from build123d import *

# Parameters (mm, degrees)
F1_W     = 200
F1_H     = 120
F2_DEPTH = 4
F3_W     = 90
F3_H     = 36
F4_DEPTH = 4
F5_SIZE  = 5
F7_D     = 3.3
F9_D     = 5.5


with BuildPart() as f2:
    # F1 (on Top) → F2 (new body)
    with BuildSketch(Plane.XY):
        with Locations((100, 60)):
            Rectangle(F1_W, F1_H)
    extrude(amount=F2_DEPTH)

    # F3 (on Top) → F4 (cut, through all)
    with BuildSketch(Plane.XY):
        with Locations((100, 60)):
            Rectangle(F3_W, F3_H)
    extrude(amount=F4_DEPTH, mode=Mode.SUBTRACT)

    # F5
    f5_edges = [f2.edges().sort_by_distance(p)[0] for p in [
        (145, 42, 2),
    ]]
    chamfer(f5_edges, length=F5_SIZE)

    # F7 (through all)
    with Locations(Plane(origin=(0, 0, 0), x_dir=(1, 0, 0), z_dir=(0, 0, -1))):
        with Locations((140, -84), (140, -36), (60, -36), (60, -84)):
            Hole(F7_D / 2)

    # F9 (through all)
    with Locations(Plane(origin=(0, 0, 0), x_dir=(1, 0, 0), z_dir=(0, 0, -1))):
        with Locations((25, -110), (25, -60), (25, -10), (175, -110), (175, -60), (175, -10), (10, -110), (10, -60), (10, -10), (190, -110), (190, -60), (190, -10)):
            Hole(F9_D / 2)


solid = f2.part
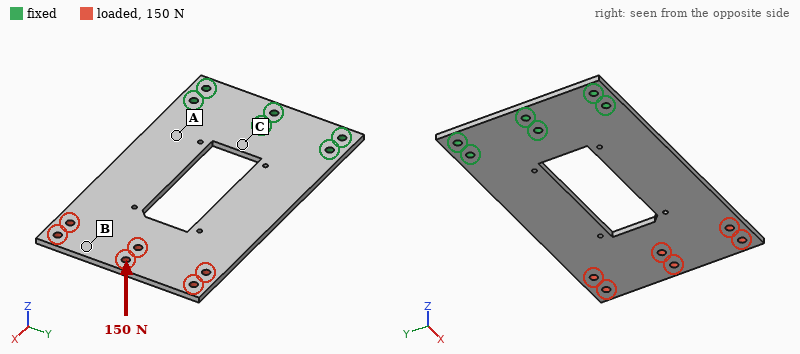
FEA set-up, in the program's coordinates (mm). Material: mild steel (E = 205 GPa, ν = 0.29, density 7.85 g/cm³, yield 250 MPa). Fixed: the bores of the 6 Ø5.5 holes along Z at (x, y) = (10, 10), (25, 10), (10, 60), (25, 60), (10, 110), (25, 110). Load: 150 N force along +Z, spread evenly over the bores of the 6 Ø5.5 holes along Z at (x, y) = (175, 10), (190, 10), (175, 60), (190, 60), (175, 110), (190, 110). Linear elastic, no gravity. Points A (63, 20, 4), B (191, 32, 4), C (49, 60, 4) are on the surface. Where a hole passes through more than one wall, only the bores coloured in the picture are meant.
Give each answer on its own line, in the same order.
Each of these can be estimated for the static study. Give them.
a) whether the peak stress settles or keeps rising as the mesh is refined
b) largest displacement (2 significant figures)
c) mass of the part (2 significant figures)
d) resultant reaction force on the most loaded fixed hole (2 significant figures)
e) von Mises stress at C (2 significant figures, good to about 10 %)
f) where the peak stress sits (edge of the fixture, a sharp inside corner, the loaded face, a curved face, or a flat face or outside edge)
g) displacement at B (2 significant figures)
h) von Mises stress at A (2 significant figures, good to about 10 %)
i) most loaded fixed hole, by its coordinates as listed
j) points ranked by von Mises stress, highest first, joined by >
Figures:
keeps rising
2.3 mm
640 g
360 N
28 MPa
edge of the fixture
2.1 mm
79 MPa
(25, 60)
A > C > B
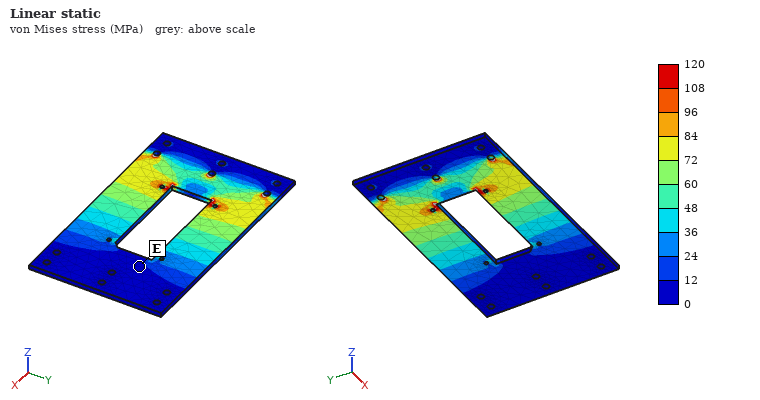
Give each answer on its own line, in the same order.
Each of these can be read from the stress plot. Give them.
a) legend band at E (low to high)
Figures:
0 to 12 MPa
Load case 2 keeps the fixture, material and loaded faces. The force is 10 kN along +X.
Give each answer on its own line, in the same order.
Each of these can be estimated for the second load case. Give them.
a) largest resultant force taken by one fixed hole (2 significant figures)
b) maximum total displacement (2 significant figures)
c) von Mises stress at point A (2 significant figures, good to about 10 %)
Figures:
2.9 kN
25 µm
28 MPa
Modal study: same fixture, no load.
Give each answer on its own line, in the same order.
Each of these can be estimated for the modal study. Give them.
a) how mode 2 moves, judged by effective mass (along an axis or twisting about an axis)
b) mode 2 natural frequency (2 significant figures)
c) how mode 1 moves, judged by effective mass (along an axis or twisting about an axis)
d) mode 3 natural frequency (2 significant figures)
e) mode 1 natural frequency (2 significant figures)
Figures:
twisting about X
320 Hz
along Z
670 Hz
99 Hz
